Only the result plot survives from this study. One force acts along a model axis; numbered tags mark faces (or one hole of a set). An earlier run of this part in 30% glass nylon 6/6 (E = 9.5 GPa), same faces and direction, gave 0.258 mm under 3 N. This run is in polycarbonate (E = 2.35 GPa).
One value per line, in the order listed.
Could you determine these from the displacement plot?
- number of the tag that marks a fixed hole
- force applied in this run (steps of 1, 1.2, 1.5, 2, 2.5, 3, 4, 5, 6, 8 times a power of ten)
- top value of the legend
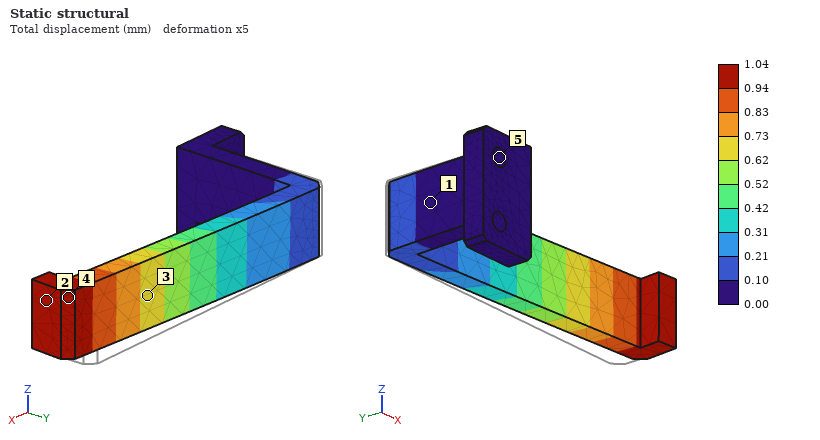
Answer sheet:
5
3 N
1.04 mm
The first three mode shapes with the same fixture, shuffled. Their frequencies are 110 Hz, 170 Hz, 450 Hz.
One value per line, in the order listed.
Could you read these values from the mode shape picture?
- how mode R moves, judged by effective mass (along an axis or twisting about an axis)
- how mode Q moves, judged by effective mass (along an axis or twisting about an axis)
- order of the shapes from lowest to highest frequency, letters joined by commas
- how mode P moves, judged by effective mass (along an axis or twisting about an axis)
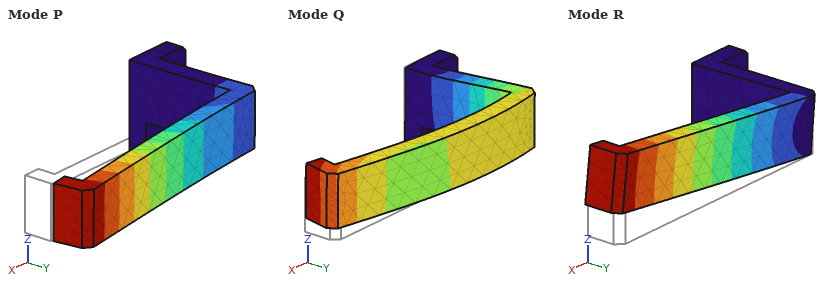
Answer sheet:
along Z
along X
P, R, Q
along Y
